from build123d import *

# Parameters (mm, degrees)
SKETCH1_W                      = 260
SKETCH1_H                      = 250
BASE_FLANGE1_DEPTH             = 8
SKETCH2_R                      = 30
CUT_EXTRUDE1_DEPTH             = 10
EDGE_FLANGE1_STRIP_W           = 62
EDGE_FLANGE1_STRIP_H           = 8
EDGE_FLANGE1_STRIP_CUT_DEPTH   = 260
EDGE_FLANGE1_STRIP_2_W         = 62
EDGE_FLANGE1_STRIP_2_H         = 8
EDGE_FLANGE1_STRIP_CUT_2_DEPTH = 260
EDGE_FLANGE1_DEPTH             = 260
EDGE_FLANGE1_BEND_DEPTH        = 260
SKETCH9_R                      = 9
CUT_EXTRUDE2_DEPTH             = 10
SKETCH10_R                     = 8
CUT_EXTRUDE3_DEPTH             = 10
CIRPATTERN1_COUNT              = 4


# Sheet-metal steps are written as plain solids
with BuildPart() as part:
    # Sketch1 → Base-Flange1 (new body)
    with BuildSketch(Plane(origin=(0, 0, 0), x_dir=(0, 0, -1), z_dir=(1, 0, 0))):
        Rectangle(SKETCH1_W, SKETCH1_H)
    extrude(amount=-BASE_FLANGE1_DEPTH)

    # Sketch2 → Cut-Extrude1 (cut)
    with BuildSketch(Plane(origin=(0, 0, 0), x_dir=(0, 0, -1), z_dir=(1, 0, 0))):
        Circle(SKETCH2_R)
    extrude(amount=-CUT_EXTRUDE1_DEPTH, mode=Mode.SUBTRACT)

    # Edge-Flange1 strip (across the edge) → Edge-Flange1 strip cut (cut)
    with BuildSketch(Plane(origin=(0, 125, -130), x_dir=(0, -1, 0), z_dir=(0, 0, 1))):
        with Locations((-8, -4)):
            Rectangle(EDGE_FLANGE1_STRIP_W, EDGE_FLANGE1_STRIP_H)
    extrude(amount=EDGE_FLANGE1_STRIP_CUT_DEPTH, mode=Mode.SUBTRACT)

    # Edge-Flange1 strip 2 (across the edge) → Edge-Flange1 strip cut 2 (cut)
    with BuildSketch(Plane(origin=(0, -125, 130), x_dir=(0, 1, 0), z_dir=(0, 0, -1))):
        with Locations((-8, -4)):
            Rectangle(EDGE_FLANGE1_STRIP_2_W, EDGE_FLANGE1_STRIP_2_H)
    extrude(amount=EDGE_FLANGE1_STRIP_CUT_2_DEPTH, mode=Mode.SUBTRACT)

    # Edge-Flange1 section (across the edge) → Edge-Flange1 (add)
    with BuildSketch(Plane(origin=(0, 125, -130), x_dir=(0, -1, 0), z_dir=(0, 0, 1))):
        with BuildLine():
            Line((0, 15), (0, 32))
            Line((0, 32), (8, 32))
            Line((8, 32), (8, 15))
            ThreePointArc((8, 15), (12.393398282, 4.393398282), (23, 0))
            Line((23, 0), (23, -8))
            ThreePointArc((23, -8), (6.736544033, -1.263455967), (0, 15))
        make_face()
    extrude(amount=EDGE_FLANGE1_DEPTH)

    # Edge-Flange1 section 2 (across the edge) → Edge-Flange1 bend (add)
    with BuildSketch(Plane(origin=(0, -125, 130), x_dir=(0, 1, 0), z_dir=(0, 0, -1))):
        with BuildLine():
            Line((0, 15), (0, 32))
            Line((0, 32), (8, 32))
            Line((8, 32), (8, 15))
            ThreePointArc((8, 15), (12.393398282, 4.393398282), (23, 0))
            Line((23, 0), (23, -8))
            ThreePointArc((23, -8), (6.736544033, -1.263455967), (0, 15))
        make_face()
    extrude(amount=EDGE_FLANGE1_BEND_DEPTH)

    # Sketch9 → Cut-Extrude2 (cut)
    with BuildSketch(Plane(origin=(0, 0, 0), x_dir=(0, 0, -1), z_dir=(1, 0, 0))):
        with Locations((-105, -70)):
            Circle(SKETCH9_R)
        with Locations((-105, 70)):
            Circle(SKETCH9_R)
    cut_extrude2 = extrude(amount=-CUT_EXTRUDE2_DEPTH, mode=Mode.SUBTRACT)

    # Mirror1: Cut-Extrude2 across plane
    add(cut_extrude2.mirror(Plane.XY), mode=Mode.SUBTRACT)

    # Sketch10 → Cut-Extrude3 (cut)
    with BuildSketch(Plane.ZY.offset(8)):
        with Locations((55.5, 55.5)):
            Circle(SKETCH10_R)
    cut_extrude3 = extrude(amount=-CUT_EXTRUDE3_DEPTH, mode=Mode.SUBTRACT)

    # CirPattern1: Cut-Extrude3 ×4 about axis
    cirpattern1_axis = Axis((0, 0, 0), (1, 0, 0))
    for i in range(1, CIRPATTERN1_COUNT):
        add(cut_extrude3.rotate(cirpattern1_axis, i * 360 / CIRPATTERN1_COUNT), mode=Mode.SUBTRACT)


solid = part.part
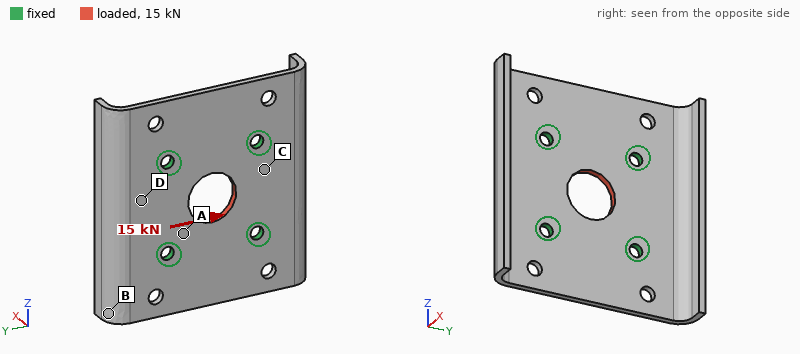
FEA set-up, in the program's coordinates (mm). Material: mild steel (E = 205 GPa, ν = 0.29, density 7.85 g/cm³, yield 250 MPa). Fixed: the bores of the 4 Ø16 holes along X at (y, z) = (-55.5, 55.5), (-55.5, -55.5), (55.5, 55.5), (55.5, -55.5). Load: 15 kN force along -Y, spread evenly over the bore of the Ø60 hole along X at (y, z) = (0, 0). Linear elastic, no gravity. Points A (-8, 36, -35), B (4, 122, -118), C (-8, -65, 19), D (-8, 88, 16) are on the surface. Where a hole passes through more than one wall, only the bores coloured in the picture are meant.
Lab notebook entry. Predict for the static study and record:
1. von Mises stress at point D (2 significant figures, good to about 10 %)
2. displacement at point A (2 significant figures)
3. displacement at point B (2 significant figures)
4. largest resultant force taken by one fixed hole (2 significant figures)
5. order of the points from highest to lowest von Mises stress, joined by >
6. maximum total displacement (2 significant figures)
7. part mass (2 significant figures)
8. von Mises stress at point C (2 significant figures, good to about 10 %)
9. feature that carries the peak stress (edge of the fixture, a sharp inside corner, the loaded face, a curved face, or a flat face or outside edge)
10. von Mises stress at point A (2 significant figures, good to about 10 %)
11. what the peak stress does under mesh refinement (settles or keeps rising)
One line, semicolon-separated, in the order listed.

3.8 MPa; 1.5 µm; 1.1 µm; 3.9 kN; A > C > D > B; 3.5 µm; 4.6 kg; 5.5 MPa; edge of the fixture; 9.7 MPa; keeps rising
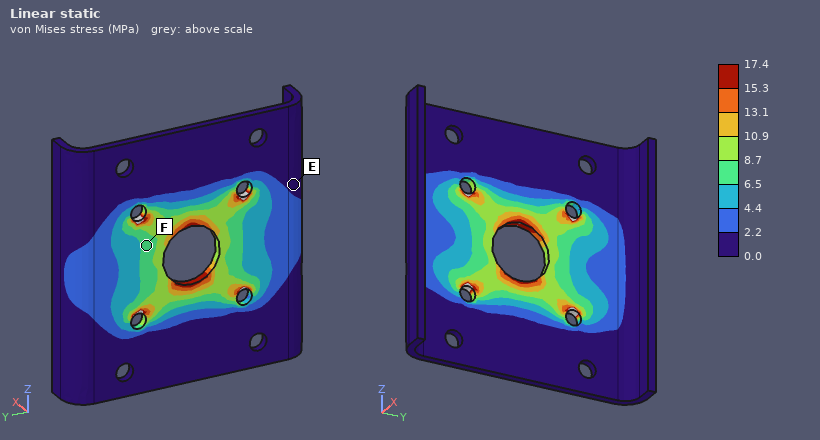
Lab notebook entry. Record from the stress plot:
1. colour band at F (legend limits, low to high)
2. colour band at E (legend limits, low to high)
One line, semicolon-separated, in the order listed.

6.5 to 8.7 MPa; 0.0 to 2.2 MPa
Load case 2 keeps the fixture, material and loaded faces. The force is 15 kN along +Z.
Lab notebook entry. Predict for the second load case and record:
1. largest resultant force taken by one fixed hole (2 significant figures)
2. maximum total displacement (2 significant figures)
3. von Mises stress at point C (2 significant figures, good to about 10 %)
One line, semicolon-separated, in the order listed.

3.9 kN; 3.4 µm; 2.7 MPa
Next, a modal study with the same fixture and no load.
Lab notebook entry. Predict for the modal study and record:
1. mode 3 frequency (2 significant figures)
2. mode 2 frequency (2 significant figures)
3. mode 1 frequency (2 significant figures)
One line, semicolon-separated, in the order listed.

860 Hz; 800 Hz; 790 Hz
